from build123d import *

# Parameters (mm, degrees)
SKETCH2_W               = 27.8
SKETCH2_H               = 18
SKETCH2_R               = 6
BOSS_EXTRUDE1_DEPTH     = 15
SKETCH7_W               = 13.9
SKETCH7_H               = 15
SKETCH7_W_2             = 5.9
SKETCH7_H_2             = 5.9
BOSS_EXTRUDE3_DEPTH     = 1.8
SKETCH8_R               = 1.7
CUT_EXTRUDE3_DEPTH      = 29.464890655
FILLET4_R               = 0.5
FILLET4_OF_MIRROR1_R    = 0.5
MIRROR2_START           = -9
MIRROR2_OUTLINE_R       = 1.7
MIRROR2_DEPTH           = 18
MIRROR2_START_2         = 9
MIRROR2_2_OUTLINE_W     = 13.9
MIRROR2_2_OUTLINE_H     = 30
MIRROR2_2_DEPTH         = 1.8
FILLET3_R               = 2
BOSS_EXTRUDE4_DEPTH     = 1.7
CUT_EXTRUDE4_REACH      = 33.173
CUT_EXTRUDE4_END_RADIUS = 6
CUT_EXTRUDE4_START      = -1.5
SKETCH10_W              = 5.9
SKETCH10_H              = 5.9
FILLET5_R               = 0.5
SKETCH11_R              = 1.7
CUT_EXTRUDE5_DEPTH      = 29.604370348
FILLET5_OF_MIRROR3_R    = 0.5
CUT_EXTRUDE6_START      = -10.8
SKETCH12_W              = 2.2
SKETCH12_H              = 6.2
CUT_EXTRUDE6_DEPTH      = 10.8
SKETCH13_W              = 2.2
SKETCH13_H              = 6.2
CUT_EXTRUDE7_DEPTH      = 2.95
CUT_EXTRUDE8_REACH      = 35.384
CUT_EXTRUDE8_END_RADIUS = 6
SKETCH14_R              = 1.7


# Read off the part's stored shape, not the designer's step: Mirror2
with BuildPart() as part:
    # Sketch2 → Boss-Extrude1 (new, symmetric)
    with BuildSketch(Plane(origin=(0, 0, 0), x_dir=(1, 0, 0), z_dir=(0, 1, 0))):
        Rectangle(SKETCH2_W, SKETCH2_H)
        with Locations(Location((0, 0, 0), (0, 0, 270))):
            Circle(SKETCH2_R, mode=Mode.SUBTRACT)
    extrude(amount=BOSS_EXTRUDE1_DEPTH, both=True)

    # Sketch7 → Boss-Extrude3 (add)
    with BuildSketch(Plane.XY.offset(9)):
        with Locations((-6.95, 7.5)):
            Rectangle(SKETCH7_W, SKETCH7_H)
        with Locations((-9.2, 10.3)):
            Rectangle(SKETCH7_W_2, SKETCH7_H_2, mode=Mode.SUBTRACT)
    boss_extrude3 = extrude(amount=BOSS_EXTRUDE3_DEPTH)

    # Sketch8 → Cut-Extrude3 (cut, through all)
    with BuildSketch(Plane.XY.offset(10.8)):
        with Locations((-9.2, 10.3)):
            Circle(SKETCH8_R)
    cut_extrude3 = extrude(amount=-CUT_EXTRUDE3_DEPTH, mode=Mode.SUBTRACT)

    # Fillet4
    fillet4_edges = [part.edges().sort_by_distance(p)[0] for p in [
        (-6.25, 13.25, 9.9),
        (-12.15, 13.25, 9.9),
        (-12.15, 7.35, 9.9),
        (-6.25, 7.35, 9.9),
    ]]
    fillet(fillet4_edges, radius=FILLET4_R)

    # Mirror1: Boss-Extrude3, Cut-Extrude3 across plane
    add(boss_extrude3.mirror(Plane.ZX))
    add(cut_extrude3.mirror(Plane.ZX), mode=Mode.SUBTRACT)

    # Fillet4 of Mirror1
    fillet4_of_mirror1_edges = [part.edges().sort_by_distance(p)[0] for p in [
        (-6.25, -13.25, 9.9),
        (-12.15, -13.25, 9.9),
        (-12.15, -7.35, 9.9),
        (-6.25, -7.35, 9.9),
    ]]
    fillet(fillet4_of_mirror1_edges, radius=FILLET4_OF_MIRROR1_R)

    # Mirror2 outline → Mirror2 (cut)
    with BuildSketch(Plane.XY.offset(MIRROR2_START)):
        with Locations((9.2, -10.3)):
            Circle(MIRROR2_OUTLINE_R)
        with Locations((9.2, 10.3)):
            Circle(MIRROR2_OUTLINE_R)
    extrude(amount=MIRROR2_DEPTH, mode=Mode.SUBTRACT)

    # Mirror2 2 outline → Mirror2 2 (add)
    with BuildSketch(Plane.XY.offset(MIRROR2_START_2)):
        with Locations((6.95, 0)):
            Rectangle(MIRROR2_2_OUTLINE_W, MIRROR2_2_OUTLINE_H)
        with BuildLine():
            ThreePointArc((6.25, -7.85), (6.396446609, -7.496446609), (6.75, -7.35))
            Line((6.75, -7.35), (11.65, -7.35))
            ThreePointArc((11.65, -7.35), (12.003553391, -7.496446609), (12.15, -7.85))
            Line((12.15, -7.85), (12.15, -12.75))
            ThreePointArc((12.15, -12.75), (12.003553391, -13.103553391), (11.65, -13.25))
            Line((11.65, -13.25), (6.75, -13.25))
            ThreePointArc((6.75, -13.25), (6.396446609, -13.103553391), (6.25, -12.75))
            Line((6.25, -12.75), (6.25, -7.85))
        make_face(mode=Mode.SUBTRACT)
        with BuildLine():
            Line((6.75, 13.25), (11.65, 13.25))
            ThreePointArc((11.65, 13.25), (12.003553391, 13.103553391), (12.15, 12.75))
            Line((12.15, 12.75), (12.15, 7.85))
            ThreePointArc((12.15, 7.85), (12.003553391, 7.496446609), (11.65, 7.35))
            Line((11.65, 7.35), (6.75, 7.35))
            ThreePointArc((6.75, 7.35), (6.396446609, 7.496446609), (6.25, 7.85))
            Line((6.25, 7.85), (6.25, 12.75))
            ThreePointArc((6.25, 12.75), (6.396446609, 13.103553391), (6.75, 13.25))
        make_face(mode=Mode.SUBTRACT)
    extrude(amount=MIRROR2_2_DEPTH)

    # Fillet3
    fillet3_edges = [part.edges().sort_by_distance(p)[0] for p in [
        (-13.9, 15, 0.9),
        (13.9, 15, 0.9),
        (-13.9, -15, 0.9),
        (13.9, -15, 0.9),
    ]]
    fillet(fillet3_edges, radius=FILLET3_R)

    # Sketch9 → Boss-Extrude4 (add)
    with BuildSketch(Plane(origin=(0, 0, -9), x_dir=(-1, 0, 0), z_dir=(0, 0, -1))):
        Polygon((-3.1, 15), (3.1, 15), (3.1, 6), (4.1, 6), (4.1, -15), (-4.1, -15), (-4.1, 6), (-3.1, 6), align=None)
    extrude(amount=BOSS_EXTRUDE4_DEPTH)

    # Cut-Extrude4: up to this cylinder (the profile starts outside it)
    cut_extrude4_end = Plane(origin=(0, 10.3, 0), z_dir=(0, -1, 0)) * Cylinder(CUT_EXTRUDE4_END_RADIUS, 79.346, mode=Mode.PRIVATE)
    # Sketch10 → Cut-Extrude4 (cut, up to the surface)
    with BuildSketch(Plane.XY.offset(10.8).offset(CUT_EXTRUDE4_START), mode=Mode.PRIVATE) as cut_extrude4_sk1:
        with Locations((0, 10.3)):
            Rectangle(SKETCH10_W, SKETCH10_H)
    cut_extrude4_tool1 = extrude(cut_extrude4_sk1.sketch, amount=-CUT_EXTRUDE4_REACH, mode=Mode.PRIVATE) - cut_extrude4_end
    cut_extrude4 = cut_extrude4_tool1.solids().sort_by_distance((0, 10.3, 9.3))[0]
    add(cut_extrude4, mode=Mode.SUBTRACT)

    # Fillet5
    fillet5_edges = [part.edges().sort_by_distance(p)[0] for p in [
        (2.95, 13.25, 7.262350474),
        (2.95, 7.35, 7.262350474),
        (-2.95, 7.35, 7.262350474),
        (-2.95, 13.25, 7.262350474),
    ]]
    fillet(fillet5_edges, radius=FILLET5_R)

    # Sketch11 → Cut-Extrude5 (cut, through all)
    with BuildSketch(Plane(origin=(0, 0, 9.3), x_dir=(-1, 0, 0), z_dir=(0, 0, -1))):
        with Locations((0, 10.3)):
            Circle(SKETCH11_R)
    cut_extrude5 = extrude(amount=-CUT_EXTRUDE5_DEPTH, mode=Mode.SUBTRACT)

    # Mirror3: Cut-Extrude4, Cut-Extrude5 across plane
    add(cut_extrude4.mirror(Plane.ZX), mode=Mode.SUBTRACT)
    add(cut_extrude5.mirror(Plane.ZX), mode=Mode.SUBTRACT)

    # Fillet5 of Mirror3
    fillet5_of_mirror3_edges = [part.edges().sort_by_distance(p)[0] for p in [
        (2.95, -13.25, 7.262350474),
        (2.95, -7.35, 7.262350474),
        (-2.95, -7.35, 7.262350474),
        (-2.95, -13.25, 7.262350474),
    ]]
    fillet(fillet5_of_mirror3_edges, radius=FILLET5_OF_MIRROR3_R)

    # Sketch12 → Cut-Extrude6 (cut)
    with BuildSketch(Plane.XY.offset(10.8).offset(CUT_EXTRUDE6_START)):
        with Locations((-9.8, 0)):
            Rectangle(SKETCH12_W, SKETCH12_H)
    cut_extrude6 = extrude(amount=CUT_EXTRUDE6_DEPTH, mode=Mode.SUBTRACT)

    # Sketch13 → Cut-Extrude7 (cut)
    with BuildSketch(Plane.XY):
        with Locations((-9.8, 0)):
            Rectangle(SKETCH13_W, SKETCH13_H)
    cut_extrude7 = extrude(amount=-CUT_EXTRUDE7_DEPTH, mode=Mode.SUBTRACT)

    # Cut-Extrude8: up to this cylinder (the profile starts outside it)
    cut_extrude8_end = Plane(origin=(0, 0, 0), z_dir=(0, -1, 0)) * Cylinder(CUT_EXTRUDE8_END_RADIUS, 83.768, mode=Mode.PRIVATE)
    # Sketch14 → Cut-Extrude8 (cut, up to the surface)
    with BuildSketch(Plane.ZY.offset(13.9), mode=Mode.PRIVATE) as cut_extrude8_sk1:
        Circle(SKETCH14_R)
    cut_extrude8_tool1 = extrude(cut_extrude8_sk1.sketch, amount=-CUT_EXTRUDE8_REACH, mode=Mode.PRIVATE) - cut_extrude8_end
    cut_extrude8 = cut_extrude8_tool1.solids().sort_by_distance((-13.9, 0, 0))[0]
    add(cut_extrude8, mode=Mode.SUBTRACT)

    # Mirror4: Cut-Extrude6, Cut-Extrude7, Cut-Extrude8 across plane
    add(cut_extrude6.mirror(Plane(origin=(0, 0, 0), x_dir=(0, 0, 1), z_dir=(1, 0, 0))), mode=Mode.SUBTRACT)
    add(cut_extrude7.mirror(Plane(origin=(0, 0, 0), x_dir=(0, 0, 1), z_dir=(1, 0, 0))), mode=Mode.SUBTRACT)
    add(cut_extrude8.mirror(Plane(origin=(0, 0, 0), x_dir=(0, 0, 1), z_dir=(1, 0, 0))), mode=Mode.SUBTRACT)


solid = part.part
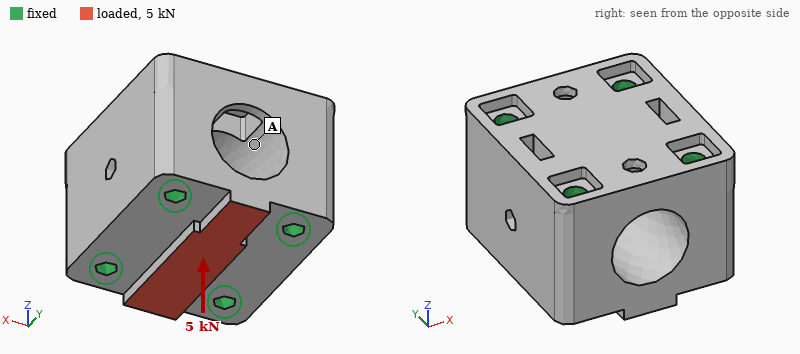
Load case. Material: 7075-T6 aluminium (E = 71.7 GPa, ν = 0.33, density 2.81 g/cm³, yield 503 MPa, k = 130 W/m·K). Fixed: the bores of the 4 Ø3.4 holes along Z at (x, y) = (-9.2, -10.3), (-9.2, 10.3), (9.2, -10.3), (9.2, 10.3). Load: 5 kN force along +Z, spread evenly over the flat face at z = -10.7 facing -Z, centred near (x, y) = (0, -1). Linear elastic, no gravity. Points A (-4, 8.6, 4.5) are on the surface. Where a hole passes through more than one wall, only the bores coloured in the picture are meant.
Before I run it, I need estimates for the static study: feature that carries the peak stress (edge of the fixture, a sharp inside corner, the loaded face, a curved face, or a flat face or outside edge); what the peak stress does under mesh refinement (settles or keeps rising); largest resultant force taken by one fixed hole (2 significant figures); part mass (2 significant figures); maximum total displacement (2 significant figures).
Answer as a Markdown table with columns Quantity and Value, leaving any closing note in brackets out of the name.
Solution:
| Quantity | Value |
|---|---|
| feature that carries the peak stress | edge of the fixture |
| what the peak stress does under mesh refinement | keeps rising |
| largest resultant force taken by one fixed hole | 1.6 kN |
| part mass | 33 g |
| maximum total displacement | 6.9 µm |
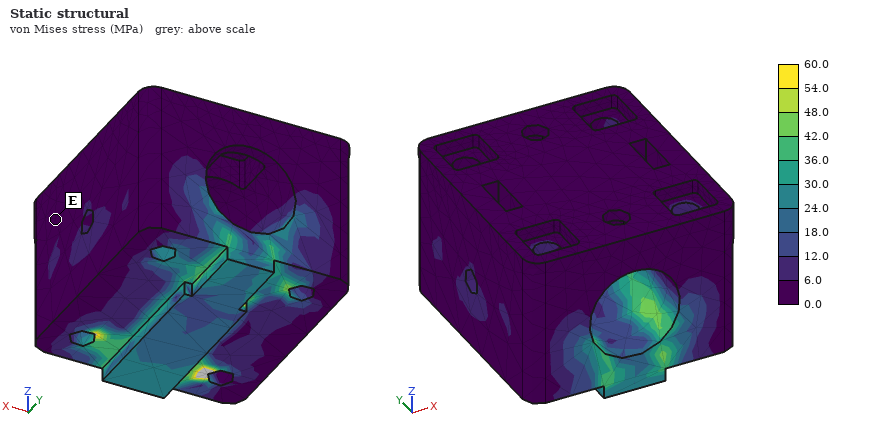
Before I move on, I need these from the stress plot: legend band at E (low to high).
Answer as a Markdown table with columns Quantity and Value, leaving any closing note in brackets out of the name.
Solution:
| Quantity | Value |
|---|---|
| legend band at E | 0.0 to 6.0 MPa |
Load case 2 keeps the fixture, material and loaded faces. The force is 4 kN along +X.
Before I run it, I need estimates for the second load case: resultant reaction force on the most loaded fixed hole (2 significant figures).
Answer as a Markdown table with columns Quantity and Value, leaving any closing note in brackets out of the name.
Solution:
| Quantity | Value |
|---|---|
| resultant reaction force on the most loaded fixed hole | 1.3 kN |
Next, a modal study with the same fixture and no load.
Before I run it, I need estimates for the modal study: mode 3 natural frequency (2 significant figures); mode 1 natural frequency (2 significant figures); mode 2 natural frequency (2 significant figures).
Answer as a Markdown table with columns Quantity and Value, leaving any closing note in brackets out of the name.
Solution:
| Quantity | Value |
|---|---|
| mode 3 natural frequency | 69 kHz |
| mode 1 natural frequency | 62 kHz |
| mode 2 natural frequency | 63 kHz |
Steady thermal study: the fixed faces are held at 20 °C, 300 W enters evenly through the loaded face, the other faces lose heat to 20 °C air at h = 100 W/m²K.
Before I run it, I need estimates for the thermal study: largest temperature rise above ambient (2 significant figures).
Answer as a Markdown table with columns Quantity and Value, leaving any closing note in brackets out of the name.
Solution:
| Quantity | Value |
|---|---|
| largest temperature rise above ambient | 87 K |
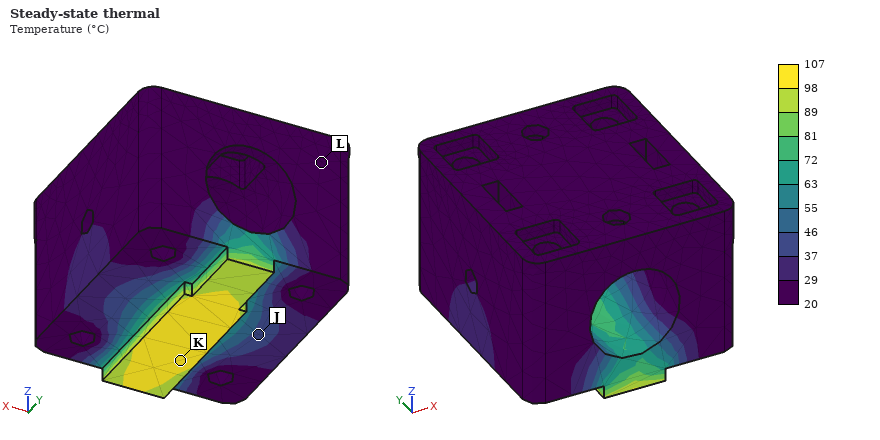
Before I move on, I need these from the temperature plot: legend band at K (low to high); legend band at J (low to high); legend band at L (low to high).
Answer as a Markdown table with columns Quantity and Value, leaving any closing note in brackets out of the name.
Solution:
| Quantity | Value |
|---|---|
| legend band at K | 98 to 107 °C |
| legend band at J | 37 to 46 °C |
| legend band at L | 20 to 29 °C |
